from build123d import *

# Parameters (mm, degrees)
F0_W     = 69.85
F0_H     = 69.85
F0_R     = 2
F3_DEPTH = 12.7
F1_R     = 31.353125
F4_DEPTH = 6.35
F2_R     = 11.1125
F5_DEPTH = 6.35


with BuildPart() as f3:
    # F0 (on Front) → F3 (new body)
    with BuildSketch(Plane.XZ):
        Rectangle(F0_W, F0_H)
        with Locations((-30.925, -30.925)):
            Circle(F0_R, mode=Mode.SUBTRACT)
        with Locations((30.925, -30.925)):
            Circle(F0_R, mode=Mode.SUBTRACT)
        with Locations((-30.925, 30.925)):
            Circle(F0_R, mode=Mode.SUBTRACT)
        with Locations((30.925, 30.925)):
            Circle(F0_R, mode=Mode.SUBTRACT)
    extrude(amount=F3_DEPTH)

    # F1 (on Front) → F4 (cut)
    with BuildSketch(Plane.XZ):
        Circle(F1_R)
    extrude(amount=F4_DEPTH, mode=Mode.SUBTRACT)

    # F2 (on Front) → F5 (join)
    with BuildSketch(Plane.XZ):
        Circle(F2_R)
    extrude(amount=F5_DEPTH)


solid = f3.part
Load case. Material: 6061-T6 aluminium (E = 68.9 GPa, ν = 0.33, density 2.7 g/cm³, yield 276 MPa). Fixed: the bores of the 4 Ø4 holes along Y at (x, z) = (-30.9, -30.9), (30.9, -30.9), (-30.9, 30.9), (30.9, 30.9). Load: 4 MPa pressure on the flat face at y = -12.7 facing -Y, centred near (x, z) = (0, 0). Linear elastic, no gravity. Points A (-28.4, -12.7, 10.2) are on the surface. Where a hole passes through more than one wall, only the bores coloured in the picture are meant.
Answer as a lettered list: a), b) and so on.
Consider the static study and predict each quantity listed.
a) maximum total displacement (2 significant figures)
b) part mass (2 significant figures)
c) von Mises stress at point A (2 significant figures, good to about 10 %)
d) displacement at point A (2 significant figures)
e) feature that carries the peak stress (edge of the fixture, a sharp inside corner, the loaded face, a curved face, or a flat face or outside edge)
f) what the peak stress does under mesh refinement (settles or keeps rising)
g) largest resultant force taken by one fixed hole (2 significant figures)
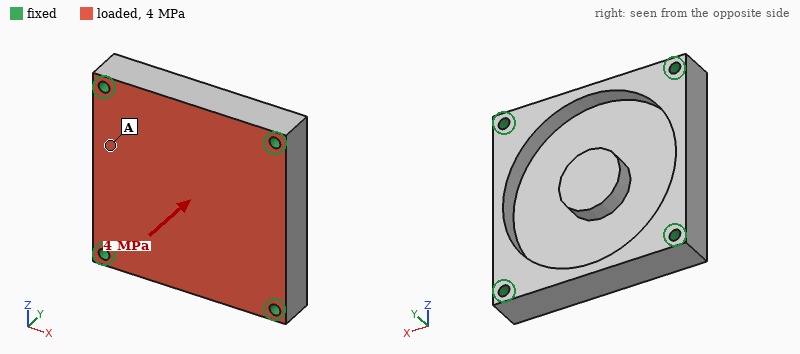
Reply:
a) 0.10 mm
b) 120 g
c) 40 MPa
d) 0.045 mm
e) edge of the fixture
f) keeps rising
g) 5.4 kN
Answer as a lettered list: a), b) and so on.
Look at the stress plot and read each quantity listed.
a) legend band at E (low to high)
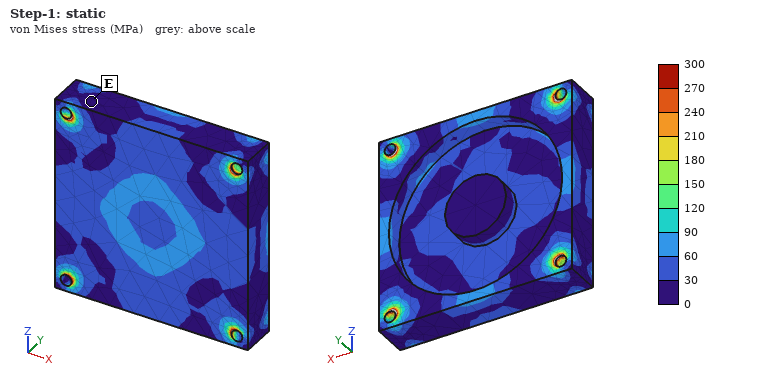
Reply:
a) 0 to 30 MPa
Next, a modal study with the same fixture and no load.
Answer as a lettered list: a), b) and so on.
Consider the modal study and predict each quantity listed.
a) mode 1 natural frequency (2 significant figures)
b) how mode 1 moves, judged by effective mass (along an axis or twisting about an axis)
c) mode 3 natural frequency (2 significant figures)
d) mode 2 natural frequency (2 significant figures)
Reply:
a) 7900 Hz
b) along Y
c) 13 kHz
d) 13 kHz
